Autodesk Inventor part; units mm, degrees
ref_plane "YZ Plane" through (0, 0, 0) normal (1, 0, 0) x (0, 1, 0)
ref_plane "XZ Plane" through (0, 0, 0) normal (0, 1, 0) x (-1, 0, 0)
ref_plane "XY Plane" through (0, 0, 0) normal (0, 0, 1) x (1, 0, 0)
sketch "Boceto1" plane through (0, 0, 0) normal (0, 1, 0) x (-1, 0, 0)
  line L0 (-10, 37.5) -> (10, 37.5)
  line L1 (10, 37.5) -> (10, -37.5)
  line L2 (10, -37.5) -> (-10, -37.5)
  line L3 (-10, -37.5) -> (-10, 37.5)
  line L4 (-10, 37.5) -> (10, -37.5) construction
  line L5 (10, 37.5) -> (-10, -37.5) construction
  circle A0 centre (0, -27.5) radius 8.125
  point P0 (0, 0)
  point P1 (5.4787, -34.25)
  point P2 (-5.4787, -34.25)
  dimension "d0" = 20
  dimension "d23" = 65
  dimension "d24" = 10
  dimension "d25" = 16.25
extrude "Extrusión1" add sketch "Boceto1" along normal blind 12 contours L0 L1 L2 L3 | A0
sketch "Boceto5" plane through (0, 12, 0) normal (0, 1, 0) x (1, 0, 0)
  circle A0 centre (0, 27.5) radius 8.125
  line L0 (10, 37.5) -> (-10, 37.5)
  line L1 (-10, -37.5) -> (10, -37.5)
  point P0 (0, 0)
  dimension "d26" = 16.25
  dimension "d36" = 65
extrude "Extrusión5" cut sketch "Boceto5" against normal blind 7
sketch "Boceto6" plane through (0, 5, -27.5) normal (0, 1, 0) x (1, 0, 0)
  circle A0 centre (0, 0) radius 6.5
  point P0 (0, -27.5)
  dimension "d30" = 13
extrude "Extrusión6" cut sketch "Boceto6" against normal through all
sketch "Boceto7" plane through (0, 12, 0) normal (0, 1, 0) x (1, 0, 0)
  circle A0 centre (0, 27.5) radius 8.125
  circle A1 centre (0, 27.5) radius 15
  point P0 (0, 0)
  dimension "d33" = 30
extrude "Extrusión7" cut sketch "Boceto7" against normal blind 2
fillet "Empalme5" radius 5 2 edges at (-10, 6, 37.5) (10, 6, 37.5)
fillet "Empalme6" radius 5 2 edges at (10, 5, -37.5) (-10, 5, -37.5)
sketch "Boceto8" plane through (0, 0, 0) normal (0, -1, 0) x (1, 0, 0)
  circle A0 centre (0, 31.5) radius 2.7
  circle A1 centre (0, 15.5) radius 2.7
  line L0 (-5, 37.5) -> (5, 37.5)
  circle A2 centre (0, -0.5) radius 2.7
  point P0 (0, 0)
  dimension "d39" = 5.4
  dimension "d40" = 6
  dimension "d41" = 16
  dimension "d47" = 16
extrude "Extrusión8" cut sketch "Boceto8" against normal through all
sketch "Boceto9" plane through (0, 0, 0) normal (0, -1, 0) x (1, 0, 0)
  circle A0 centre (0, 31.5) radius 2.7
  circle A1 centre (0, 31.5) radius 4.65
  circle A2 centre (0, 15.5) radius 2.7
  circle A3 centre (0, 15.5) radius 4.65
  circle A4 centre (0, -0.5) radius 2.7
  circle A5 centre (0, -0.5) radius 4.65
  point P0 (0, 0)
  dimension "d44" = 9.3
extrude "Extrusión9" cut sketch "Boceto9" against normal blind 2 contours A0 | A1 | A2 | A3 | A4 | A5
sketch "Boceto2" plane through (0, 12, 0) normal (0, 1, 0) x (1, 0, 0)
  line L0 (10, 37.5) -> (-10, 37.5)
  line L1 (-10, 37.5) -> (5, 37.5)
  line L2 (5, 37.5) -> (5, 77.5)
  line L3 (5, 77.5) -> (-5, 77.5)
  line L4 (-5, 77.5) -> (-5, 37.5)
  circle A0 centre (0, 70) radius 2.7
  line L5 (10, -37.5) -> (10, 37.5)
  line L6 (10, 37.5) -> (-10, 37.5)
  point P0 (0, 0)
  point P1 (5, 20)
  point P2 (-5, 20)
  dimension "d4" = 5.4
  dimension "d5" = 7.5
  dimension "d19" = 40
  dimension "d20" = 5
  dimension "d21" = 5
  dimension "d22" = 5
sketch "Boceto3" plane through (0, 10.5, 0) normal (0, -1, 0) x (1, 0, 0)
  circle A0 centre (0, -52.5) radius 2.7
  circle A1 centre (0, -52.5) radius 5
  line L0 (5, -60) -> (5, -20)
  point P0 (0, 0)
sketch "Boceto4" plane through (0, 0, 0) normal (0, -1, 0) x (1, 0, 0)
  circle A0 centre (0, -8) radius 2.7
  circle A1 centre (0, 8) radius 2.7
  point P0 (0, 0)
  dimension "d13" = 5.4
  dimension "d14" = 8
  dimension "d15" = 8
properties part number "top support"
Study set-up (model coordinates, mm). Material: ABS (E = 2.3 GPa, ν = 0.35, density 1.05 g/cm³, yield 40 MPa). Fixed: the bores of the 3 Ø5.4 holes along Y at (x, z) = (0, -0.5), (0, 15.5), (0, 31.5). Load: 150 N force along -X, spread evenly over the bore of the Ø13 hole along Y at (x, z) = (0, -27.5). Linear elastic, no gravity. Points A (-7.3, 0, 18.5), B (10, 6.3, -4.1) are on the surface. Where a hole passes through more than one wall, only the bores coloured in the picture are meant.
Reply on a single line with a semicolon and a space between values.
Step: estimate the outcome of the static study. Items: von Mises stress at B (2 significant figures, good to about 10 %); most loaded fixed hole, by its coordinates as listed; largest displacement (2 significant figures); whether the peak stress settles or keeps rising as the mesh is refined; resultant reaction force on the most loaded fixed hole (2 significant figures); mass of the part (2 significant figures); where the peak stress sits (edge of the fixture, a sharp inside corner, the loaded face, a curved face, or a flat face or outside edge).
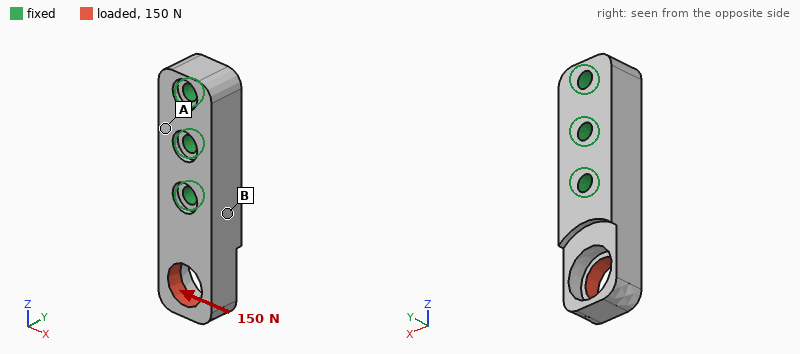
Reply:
4.5 MPa; (0, -0.5); 0.28 mm; keeps rising; 280 N; 15 g; edge of the fixture
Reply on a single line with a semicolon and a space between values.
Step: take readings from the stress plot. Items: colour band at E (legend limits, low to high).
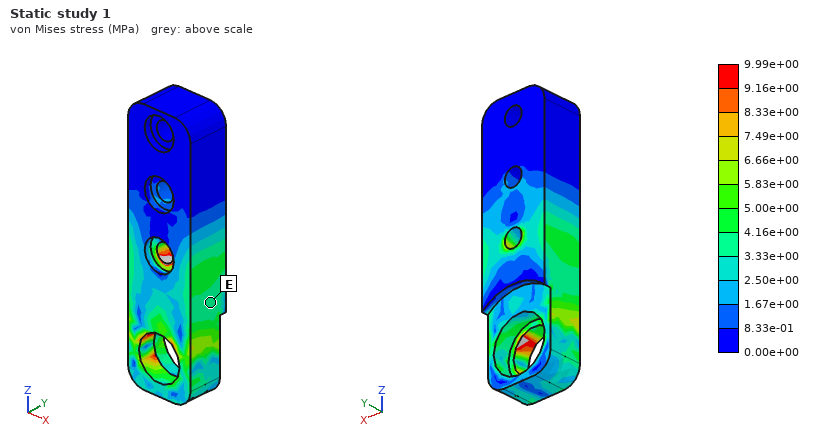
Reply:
3.33e+00 to 4.16e+00 MPa
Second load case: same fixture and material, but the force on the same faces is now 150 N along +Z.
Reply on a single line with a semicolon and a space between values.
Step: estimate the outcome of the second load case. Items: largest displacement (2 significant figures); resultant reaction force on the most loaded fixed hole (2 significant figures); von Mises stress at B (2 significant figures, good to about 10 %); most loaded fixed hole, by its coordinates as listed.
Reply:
92 µm; 120 N; 0.47 MPa; (0, -0.5)
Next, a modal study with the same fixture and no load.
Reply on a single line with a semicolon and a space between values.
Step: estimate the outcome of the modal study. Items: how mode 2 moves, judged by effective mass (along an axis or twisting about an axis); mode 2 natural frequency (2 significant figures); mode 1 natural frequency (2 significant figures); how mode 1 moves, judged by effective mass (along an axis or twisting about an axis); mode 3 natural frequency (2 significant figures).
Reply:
along X; 2700 Hz; 2300 Hz; along Y; 4500 Hz
